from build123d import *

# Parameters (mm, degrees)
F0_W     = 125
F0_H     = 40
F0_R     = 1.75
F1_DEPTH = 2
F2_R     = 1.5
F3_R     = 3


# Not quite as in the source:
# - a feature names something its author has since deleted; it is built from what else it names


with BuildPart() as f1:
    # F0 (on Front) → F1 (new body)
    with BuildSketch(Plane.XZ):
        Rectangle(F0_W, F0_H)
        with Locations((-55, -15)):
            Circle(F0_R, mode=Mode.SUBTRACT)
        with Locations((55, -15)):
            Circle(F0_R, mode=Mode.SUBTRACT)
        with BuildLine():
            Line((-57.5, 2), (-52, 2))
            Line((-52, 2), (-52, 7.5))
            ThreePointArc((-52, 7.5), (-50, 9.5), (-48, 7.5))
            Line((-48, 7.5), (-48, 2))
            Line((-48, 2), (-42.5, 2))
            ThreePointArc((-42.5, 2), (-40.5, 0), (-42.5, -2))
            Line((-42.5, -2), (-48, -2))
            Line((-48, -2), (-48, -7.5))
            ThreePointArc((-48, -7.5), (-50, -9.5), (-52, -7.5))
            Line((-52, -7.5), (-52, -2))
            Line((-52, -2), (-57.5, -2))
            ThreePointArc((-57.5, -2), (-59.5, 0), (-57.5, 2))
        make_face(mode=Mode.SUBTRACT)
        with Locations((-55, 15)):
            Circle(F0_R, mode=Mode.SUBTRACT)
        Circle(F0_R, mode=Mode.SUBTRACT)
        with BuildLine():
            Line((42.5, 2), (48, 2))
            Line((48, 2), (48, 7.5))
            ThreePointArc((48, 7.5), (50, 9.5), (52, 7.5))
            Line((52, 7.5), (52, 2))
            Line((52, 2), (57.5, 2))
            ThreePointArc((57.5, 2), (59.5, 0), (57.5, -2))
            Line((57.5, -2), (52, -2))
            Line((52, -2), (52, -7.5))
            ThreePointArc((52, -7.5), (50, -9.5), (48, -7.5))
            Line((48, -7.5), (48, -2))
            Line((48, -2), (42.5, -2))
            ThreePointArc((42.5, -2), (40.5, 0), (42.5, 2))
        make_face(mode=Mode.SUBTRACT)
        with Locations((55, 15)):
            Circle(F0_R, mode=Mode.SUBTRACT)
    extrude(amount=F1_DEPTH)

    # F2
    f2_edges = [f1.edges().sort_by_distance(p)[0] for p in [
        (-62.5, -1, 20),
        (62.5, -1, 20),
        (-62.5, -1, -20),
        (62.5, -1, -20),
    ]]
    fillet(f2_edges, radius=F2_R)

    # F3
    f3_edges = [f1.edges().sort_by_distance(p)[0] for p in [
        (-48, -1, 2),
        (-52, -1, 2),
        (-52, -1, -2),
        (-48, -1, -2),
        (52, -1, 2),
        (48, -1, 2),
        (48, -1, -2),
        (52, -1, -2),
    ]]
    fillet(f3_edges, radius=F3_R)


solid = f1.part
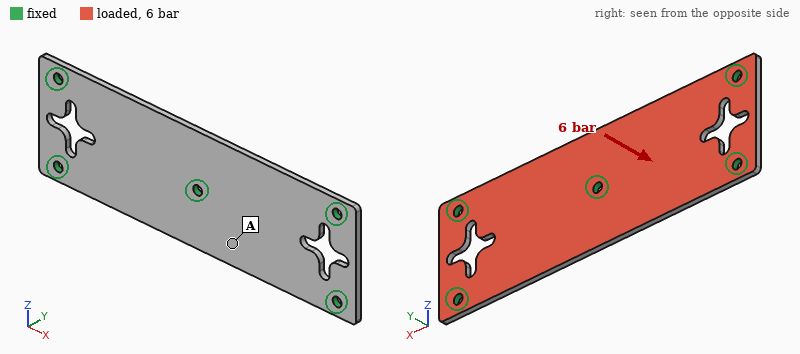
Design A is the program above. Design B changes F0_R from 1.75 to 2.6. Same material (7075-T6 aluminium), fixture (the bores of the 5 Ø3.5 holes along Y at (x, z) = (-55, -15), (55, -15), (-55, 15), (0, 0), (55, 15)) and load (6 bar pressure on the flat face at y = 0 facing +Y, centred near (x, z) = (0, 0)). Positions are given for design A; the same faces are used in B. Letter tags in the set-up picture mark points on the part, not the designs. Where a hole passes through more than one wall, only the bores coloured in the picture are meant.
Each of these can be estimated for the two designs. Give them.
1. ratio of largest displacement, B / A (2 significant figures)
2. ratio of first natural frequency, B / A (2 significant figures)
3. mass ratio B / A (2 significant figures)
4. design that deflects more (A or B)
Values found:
0.89
1.1
0.99
A
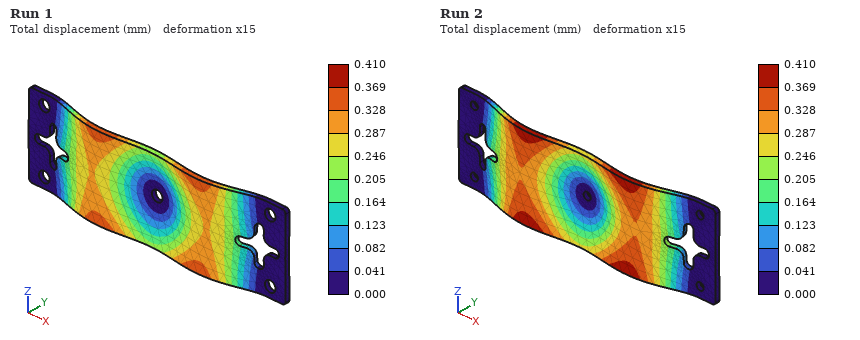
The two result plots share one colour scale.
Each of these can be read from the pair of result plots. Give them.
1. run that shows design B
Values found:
Run 1
